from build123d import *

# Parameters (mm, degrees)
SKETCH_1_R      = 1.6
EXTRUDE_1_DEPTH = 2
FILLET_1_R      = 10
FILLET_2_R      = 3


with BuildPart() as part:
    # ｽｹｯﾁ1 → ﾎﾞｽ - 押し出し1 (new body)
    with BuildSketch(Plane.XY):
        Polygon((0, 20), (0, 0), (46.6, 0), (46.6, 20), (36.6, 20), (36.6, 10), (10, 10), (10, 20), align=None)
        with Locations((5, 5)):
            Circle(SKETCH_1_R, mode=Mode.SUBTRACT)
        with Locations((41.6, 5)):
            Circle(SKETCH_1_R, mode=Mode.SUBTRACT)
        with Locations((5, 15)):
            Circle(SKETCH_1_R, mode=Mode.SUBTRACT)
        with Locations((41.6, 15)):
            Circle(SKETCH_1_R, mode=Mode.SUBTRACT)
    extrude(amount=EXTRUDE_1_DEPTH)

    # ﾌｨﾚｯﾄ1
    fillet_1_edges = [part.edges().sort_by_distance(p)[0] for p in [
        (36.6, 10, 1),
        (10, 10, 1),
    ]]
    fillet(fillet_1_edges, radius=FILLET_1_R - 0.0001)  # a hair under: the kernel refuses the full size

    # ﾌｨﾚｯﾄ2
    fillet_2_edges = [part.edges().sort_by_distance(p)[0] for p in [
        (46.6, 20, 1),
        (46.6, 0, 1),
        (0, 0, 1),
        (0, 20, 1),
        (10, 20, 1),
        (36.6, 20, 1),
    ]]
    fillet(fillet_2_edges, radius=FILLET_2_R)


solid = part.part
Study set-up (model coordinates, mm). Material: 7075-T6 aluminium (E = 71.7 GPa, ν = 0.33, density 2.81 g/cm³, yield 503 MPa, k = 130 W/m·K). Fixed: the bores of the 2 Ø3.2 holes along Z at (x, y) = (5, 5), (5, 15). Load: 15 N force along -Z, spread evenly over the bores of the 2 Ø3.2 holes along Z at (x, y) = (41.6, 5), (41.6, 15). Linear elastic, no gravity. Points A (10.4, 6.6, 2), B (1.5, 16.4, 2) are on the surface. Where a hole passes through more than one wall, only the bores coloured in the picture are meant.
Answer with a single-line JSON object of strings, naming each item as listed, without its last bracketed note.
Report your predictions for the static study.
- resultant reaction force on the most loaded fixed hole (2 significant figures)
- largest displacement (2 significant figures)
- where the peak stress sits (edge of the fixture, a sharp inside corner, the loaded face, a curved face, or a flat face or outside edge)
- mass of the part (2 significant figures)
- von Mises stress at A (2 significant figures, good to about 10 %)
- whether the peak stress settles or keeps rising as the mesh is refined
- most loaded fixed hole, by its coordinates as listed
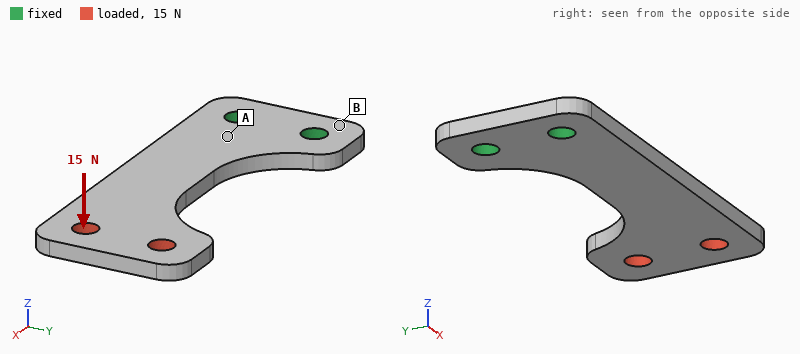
{"resultant reaction force on the most loaded fixed hole": "11 N", "largest displacement": "0.50 mm", "where the peak stress sits": "edge of the fixture", "mass of the part": "3.7 g", "von Mises stress at A": "47 MPa", "whether the peak stress settles or keeps rising as the mesh is refined": "keeps rising", "most loaded fixed hole, by its coordinates as listed": "(5, 5)"}
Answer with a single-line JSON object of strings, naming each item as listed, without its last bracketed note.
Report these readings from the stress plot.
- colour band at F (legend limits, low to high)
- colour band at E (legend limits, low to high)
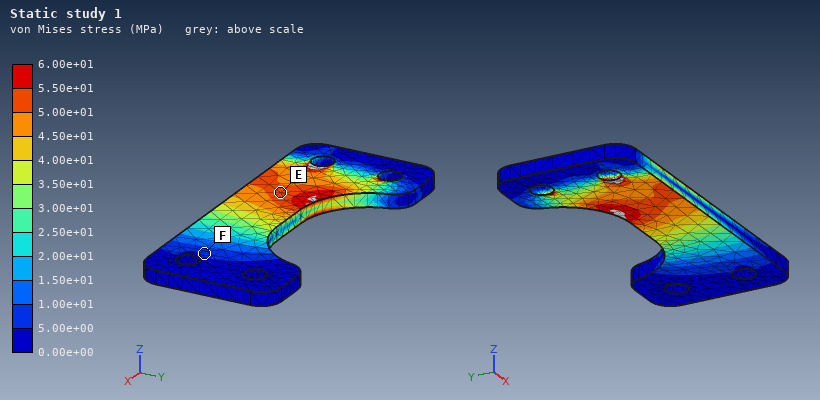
{"colour band at F": "5.00e+00 to 1.00e+01 MPa", "colour band at E": "5.00e+01 to 5.50e+01 MPa"}
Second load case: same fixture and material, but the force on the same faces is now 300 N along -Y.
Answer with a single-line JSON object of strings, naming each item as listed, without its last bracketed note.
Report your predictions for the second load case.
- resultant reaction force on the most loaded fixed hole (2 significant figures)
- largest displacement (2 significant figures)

{"resultant reaction force on the most loaded fixed hole": "1.0 kN", "largest displacement": "0.36 mm"}
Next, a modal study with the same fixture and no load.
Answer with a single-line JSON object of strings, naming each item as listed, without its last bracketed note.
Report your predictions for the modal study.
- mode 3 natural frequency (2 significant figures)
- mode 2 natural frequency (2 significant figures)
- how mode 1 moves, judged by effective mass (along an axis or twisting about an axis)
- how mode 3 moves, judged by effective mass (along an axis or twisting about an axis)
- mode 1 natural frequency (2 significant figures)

{"mode 3 natural frequency": "4500 Hz", "mode 2 natural frequency": "3600 Hz", "how mode 1 moves, judged by effective mass": "along Z", "how mode 3 moves, judged by effective mass": "along Y", "mode 1 natural frequency": "860 Hz"}
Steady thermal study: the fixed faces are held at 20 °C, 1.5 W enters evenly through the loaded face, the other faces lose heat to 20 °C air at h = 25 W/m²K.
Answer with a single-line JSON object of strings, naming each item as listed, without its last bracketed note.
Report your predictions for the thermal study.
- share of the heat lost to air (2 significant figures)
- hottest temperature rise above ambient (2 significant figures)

{"share of the heat lost to air": "20 %", "hottest temperature rise above ambient": "16 K"}
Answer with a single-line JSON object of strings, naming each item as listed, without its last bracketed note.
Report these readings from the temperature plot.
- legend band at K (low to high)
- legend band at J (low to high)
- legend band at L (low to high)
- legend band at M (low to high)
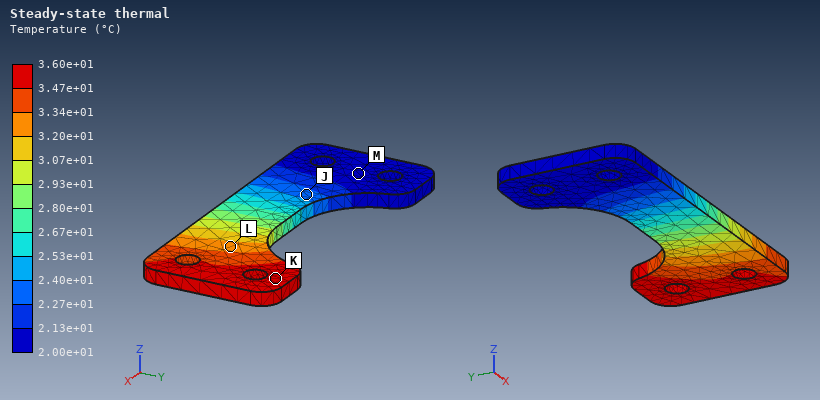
{"legend band at K": "3.47e+01 to 3.60e+01 °C", "legend band at J": "2.27e+01 to 2.40e+01 °C", "legend band at L": "3.20e+01 to 3.34e+01 °C", "legend band at M": "2.00e+01 to 2.13e+01 °C"}
